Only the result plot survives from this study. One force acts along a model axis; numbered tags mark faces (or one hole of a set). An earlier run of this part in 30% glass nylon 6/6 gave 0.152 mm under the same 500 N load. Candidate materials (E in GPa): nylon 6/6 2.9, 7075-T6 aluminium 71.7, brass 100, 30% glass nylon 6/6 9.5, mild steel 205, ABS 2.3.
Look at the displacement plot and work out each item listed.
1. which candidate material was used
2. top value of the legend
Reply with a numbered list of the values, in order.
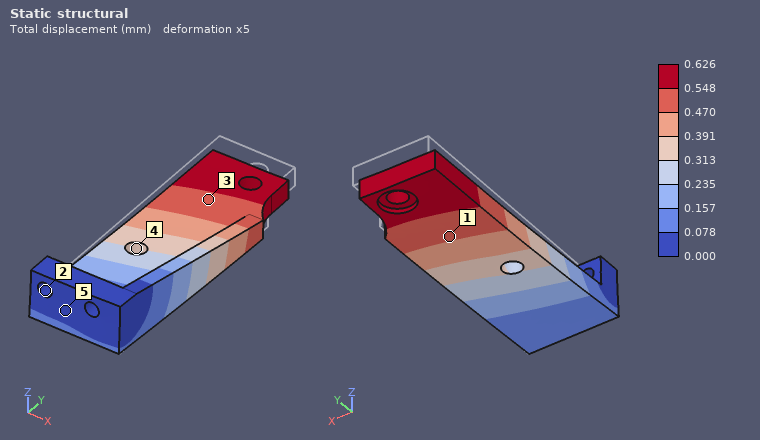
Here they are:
1. ABS
2. 0.626 mm
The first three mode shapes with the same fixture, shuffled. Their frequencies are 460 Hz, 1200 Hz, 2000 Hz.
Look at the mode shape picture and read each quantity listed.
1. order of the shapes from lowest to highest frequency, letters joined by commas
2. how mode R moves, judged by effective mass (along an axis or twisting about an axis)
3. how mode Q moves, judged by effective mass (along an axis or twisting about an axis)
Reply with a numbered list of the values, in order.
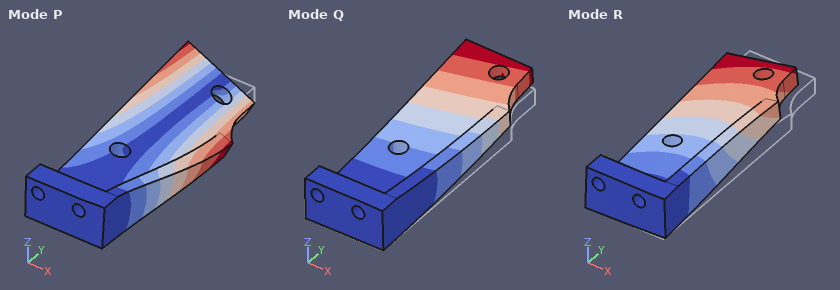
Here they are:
1. Q, R, P
2. along X
3. along Z
